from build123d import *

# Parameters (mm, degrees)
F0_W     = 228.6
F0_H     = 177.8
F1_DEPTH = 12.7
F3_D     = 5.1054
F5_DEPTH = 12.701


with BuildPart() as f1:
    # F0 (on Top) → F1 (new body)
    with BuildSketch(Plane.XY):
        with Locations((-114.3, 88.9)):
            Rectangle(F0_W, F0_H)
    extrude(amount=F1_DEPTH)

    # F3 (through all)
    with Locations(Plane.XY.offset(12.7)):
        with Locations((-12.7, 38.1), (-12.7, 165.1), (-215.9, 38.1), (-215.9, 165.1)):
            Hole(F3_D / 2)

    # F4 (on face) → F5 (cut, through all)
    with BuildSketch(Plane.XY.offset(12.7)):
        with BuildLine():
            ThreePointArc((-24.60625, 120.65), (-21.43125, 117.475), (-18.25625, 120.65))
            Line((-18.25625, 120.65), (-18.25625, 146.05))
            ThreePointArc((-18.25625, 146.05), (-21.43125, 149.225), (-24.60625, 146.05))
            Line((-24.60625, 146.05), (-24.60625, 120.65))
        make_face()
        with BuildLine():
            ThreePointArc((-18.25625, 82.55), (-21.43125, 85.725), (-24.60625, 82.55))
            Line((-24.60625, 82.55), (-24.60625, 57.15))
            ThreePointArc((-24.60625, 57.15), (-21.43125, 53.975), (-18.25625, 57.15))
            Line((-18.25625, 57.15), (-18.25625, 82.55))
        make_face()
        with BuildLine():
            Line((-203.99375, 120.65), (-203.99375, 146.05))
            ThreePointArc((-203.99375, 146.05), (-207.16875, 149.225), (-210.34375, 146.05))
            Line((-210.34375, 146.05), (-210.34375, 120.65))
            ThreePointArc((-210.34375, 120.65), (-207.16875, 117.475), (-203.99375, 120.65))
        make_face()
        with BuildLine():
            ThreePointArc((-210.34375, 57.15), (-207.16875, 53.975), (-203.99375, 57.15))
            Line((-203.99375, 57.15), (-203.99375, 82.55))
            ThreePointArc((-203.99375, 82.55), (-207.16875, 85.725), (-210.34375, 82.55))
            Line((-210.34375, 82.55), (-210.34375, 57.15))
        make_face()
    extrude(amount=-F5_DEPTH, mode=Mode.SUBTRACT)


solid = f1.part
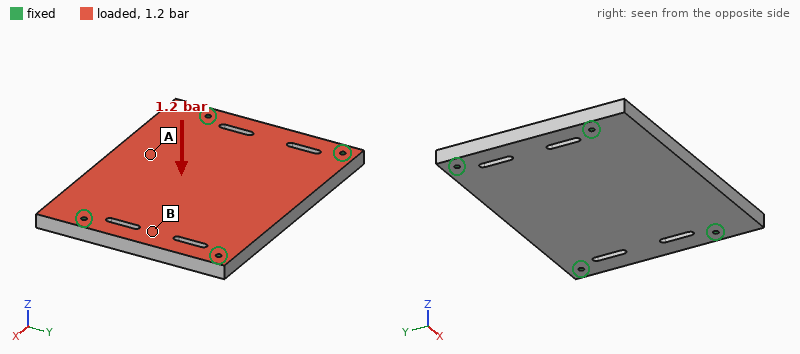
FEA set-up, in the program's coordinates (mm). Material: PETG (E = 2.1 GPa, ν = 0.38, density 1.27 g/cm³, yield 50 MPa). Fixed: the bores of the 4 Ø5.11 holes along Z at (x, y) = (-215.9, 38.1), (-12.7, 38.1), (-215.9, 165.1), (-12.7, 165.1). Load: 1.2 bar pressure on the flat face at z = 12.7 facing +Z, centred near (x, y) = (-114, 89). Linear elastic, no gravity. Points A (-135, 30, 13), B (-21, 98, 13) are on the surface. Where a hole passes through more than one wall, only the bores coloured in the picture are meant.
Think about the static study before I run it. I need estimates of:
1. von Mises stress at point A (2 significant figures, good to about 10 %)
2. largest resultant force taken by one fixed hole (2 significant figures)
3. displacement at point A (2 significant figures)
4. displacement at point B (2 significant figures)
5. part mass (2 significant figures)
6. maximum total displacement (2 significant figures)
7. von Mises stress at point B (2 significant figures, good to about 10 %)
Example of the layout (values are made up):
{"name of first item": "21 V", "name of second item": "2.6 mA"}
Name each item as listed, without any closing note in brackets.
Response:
{"von Mises stress at point A": "9.6 MPa", "largest resultant force taken by one fixed hole": "1.4 kN", "displacement at point A": "2.5 mm", "displacement at point B": "0.70 mm", "part mass": "640 g", "maximum total displacement": "2.9 mm", "von Mises stress at point B": "4.6 MPa"}
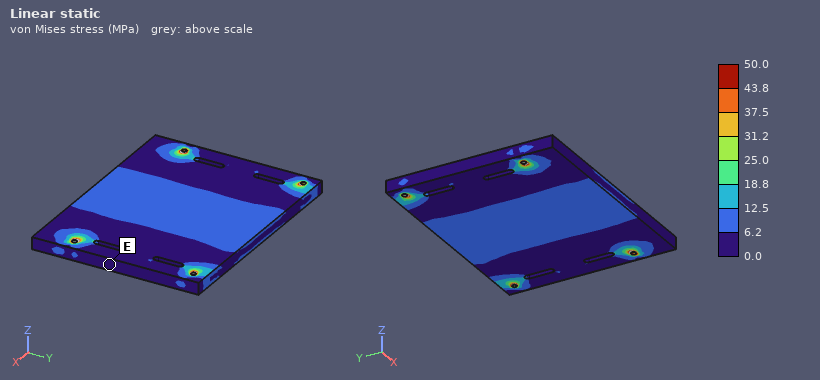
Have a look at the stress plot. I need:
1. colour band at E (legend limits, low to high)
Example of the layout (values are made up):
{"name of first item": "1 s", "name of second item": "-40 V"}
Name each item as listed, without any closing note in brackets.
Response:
{"colour band at E": "0.0 to 6.2 MPa"}
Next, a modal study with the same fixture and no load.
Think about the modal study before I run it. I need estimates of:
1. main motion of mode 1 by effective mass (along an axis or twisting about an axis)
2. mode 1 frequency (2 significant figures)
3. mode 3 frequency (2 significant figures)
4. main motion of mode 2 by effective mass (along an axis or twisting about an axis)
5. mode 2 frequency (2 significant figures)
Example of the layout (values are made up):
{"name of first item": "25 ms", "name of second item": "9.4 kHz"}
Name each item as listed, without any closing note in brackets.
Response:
{"main motion of mode 1 by effective mass": "along Z", "mode 1 frequency": "300 Hz", "mode 3 frequency": "710 Hz", "main motion of mode 2 by effective mass": "twisting about X", "mode 2 frequency": "410 Hz"}
